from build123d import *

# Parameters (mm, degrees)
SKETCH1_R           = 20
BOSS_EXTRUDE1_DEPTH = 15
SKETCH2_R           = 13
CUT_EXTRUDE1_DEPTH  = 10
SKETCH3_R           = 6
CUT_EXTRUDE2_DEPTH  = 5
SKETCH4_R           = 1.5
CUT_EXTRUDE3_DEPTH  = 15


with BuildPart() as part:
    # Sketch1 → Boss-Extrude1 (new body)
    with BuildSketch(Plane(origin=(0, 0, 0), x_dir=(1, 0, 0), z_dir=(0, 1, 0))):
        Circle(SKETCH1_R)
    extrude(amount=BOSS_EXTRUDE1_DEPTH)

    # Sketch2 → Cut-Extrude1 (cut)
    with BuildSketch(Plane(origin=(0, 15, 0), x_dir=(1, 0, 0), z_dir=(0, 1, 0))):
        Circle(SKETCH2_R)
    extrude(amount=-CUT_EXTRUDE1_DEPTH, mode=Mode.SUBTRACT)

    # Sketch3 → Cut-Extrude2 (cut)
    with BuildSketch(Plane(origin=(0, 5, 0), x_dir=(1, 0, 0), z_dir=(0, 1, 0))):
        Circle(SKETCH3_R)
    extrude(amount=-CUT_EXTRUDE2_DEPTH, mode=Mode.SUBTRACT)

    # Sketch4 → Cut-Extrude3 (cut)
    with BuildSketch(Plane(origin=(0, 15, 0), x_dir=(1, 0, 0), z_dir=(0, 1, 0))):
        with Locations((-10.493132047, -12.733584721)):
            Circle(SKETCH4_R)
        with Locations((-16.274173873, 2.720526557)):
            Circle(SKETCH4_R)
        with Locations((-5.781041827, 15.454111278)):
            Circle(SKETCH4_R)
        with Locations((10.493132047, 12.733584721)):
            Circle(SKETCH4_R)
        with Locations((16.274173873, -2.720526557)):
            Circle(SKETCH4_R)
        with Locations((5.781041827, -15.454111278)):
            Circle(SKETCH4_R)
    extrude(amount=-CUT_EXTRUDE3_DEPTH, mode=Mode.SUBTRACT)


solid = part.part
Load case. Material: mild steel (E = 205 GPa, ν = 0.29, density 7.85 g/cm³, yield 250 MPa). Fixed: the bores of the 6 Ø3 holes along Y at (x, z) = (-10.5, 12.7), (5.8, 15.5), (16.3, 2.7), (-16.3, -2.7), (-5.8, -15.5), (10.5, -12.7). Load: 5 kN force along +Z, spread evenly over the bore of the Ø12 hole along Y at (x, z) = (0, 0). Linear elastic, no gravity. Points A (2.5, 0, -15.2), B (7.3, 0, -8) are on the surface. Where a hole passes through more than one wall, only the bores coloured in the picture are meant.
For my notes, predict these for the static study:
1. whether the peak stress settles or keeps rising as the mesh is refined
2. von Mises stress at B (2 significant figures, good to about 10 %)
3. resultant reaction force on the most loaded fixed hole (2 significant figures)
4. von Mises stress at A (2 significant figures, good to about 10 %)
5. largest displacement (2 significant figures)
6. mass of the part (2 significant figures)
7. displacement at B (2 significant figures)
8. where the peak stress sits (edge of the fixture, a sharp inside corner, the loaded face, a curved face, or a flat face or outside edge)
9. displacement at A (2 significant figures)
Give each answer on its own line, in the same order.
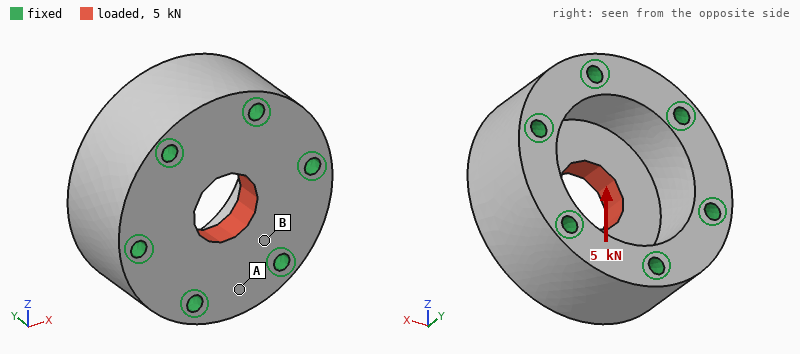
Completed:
keeps rising
23 MPa
1.2 kN
6.0 MPa
1.5 µm
97 g
0.64 µm
edge of the fixture
0.74 µm
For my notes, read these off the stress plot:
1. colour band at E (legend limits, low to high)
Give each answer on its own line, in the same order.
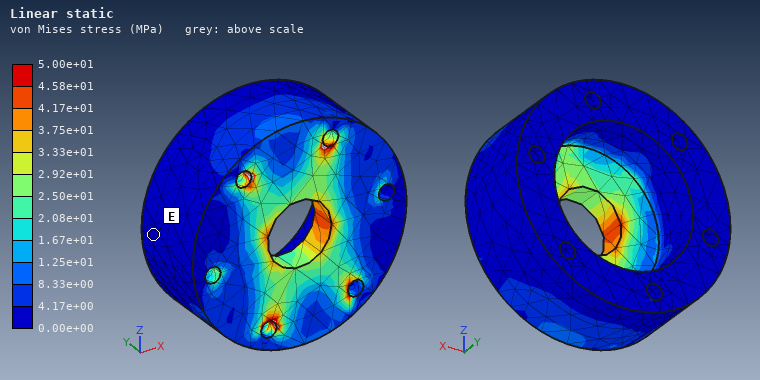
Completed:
0.00e+00 to 4.17e+00 MPa
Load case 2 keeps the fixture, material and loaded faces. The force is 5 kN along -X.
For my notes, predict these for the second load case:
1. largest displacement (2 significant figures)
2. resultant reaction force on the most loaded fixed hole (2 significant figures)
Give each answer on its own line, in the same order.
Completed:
1.5 µm
1.2 kN
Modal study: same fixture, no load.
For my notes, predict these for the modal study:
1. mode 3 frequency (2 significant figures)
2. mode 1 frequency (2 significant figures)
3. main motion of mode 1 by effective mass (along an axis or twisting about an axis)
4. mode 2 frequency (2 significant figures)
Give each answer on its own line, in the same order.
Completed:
68 kHz
54 kHz
along Y
68 kHz
